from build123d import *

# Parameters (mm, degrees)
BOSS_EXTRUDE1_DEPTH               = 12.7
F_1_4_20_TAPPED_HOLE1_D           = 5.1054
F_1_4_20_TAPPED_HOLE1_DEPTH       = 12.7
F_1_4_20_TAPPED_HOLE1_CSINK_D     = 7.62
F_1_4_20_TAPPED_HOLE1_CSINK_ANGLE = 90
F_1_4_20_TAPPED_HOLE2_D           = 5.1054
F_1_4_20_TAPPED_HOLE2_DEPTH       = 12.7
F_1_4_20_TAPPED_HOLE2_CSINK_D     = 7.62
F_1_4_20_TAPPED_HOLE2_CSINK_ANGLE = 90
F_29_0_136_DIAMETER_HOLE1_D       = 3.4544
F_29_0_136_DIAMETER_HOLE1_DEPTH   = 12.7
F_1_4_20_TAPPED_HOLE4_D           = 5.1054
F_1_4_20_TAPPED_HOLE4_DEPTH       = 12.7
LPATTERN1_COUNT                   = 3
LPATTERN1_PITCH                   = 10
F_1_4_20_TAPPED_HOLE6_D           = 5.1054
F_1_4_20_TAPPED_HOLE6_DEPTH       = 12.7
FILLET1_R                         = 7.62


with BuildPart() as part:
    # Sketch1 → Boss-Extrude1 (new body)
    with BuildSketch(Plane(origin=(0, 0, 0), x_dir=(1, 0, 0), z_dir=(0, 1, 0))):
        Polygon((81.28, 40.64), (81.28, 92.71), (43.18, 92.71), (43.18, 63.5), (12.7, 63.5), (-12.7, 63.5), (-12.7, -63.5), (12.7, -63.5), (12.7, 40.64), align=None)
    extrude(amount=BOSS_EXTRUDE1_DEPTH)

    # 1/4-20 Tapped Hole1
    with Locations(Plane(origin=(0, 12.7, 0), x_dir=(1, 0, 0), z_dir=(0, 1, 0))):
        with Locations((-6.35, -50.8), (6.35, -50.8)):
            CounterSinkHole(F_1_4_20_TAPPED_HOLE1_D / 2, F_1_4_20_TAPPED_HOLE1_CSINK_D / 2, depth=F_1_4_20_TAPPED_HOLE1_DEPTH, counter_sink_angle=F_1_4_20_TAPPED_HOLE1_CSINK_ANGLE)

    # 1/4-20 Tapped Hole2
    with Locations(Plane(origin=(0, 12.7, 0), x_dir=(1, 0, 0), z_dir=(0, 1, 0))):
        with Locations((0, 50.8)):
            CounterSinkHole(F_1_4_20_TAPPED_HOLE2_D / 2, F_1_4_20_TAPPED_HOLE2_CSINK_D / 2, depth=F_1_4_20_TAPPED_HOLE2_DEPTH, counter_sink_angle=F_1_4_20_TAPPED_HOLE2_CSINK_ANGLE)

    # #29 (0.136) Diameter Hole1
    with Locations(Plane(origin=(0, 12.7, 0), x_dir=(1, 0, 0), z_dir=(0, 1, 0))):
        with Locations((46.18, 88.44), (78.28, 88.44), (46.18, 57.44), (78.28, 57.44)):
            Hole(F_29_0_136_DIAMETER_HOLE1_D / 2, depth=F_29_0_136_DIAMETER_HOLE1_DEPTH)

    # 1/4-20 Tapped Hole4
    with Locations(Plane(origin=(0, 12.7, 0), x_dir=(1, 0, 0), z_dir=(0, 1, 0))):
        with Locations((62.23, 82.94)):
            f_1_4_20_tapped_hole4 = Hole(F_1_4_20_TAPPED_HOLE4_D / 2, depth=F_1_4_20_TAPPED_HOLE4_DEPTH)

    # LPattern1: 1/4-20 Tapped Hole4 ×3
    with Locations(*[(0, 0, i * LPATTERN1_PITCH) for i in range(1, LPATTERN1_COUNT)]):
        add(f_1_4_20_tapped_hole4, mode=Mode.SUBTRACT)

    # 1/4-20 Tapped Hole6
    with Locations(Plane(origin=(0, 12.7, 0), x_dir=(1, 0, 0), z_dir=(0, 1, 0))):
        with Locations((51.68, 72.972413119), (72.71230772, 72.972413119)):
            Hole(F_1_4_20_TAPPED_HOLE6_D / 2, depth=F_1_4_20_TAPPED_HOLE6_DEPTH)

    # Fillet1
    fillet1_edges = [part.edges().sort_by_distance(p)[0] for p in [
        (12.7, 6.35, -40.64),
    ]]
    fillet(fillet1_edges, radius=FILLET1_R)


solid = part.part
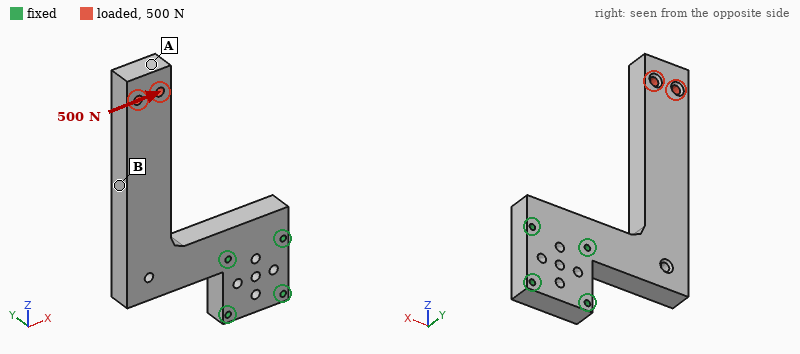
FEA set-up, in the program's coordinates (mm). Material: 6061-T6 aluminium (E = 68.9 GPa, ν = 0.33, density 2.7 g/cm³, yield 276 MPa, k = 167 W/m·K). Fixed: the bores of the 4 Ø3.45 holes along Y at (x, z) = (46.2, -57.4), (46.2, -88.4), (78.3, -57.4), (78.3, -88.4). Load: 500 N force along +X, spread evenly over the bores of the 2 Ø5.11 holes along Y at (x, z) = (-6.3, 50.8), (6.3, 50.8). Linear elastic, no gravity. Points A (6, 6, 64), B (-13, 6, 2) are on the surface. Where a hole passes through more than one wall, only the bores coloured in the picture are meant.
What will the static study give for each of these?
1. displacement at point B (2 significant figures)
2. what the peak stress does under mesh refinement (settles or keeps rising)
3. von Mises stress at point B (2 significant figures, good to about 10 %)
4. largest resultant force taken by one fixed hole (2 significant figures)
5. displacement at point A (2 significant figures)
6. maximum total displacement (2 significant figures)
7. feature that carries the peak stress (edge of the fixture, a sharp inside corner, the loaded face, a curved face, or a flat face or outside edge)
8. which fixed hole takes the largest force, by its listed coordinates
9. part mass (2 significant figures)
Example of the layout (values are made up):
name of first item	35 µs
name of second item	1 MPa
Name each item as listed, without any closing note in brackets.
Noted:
displacement at point B	0.25 mm
what the peak stress does under mesh refinement	keeps rising
von Mises stress at point B	18 MPa
largest resultant force taken by one fixed hole	1.7 kN
displacement at point A	0.50 mm
maximum total displacement	0.52 mm
feature that carries the peak stress	edge of the fixture
which fixed hole takes the largest force, by its listed coordinates	(78.3, -57.4)
part mass	200 g
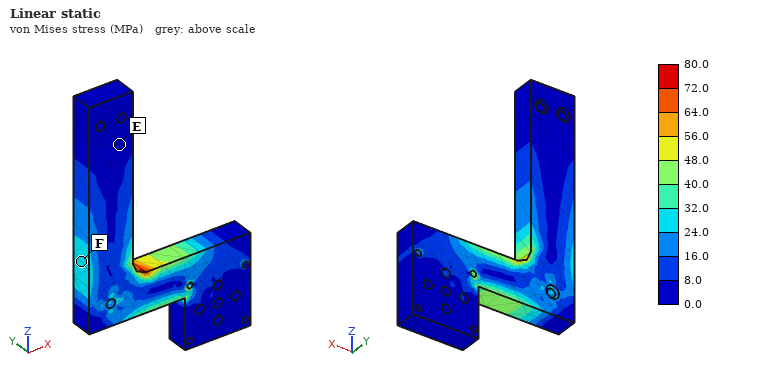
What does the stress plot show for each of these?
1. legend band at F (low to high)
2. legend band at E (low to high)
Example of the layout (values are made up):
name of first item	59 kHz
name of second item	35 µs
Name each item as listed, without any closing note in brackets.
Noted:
legend band at F	24.0 to 32.0 MPa
legend band at E	0.0 to 8.0 MPa
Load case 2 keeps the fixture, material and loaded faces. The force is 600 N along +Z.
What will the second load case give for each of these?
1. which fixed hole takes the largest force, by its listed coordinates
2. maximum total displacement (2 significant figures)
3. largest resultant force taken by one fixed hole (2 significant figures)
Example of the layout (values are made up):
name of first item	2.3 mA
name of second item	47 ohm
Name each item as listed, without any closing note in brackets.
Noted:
which fixed hole takes the largest force, by its listed coordinates	(46.2, -57.4)
maximum total displacement	0.13 mm
largest resultant force taken by one fixed hole	1.3 kN
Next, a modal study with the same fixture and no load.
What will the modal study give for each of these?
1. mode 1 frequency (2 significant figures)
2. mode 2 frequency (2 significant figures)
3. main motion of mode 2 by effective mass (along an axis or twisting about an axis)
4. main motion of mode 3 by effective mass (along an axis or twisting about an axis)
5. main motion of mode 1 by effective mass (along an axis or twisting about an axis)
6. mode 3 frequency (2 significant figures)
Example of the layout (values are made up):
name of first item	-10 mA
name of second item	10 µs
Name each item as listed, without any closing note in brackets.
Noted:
mode 1 frequency	470 Hz
mode 2 frequency	810 Hz
main motion of mode 2 by effective mass	along X
main motion of mode 3 by effective mass	along Y
main motion of mode 1 by effective mass	along Y
mode 3 frequency	1800 Hz
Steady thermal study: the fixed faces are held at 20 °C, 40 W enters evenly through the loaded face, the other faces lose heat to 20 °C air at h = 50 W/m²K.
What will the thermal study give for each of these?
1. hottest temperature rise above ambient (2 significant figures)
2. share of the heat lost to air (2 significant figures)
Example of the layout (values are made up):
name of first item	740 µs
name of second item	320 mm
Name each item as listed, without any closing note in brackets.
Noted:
hottest temperature rise above ambient	68 K
share of the heat lost to air	52 %
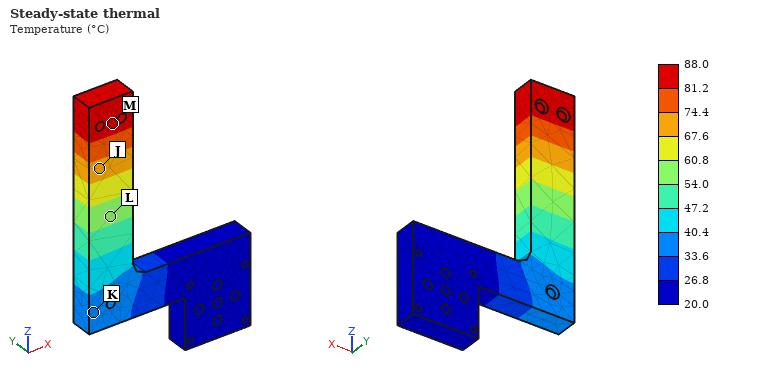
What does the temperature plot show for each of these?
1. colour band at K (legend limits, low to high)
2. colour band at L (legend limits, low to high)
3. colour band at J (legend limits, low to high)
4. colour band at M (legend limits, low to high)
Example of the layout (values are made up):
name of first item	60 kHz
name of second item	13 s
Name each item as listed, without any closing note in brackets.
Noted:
colour band at K	33.6 to 40.4 °C
colour band at L	54.0 to 60.8 °C
colour band at J	67.6 to 74.4 °C
colour band at M	81.2 to 88.0 °C
